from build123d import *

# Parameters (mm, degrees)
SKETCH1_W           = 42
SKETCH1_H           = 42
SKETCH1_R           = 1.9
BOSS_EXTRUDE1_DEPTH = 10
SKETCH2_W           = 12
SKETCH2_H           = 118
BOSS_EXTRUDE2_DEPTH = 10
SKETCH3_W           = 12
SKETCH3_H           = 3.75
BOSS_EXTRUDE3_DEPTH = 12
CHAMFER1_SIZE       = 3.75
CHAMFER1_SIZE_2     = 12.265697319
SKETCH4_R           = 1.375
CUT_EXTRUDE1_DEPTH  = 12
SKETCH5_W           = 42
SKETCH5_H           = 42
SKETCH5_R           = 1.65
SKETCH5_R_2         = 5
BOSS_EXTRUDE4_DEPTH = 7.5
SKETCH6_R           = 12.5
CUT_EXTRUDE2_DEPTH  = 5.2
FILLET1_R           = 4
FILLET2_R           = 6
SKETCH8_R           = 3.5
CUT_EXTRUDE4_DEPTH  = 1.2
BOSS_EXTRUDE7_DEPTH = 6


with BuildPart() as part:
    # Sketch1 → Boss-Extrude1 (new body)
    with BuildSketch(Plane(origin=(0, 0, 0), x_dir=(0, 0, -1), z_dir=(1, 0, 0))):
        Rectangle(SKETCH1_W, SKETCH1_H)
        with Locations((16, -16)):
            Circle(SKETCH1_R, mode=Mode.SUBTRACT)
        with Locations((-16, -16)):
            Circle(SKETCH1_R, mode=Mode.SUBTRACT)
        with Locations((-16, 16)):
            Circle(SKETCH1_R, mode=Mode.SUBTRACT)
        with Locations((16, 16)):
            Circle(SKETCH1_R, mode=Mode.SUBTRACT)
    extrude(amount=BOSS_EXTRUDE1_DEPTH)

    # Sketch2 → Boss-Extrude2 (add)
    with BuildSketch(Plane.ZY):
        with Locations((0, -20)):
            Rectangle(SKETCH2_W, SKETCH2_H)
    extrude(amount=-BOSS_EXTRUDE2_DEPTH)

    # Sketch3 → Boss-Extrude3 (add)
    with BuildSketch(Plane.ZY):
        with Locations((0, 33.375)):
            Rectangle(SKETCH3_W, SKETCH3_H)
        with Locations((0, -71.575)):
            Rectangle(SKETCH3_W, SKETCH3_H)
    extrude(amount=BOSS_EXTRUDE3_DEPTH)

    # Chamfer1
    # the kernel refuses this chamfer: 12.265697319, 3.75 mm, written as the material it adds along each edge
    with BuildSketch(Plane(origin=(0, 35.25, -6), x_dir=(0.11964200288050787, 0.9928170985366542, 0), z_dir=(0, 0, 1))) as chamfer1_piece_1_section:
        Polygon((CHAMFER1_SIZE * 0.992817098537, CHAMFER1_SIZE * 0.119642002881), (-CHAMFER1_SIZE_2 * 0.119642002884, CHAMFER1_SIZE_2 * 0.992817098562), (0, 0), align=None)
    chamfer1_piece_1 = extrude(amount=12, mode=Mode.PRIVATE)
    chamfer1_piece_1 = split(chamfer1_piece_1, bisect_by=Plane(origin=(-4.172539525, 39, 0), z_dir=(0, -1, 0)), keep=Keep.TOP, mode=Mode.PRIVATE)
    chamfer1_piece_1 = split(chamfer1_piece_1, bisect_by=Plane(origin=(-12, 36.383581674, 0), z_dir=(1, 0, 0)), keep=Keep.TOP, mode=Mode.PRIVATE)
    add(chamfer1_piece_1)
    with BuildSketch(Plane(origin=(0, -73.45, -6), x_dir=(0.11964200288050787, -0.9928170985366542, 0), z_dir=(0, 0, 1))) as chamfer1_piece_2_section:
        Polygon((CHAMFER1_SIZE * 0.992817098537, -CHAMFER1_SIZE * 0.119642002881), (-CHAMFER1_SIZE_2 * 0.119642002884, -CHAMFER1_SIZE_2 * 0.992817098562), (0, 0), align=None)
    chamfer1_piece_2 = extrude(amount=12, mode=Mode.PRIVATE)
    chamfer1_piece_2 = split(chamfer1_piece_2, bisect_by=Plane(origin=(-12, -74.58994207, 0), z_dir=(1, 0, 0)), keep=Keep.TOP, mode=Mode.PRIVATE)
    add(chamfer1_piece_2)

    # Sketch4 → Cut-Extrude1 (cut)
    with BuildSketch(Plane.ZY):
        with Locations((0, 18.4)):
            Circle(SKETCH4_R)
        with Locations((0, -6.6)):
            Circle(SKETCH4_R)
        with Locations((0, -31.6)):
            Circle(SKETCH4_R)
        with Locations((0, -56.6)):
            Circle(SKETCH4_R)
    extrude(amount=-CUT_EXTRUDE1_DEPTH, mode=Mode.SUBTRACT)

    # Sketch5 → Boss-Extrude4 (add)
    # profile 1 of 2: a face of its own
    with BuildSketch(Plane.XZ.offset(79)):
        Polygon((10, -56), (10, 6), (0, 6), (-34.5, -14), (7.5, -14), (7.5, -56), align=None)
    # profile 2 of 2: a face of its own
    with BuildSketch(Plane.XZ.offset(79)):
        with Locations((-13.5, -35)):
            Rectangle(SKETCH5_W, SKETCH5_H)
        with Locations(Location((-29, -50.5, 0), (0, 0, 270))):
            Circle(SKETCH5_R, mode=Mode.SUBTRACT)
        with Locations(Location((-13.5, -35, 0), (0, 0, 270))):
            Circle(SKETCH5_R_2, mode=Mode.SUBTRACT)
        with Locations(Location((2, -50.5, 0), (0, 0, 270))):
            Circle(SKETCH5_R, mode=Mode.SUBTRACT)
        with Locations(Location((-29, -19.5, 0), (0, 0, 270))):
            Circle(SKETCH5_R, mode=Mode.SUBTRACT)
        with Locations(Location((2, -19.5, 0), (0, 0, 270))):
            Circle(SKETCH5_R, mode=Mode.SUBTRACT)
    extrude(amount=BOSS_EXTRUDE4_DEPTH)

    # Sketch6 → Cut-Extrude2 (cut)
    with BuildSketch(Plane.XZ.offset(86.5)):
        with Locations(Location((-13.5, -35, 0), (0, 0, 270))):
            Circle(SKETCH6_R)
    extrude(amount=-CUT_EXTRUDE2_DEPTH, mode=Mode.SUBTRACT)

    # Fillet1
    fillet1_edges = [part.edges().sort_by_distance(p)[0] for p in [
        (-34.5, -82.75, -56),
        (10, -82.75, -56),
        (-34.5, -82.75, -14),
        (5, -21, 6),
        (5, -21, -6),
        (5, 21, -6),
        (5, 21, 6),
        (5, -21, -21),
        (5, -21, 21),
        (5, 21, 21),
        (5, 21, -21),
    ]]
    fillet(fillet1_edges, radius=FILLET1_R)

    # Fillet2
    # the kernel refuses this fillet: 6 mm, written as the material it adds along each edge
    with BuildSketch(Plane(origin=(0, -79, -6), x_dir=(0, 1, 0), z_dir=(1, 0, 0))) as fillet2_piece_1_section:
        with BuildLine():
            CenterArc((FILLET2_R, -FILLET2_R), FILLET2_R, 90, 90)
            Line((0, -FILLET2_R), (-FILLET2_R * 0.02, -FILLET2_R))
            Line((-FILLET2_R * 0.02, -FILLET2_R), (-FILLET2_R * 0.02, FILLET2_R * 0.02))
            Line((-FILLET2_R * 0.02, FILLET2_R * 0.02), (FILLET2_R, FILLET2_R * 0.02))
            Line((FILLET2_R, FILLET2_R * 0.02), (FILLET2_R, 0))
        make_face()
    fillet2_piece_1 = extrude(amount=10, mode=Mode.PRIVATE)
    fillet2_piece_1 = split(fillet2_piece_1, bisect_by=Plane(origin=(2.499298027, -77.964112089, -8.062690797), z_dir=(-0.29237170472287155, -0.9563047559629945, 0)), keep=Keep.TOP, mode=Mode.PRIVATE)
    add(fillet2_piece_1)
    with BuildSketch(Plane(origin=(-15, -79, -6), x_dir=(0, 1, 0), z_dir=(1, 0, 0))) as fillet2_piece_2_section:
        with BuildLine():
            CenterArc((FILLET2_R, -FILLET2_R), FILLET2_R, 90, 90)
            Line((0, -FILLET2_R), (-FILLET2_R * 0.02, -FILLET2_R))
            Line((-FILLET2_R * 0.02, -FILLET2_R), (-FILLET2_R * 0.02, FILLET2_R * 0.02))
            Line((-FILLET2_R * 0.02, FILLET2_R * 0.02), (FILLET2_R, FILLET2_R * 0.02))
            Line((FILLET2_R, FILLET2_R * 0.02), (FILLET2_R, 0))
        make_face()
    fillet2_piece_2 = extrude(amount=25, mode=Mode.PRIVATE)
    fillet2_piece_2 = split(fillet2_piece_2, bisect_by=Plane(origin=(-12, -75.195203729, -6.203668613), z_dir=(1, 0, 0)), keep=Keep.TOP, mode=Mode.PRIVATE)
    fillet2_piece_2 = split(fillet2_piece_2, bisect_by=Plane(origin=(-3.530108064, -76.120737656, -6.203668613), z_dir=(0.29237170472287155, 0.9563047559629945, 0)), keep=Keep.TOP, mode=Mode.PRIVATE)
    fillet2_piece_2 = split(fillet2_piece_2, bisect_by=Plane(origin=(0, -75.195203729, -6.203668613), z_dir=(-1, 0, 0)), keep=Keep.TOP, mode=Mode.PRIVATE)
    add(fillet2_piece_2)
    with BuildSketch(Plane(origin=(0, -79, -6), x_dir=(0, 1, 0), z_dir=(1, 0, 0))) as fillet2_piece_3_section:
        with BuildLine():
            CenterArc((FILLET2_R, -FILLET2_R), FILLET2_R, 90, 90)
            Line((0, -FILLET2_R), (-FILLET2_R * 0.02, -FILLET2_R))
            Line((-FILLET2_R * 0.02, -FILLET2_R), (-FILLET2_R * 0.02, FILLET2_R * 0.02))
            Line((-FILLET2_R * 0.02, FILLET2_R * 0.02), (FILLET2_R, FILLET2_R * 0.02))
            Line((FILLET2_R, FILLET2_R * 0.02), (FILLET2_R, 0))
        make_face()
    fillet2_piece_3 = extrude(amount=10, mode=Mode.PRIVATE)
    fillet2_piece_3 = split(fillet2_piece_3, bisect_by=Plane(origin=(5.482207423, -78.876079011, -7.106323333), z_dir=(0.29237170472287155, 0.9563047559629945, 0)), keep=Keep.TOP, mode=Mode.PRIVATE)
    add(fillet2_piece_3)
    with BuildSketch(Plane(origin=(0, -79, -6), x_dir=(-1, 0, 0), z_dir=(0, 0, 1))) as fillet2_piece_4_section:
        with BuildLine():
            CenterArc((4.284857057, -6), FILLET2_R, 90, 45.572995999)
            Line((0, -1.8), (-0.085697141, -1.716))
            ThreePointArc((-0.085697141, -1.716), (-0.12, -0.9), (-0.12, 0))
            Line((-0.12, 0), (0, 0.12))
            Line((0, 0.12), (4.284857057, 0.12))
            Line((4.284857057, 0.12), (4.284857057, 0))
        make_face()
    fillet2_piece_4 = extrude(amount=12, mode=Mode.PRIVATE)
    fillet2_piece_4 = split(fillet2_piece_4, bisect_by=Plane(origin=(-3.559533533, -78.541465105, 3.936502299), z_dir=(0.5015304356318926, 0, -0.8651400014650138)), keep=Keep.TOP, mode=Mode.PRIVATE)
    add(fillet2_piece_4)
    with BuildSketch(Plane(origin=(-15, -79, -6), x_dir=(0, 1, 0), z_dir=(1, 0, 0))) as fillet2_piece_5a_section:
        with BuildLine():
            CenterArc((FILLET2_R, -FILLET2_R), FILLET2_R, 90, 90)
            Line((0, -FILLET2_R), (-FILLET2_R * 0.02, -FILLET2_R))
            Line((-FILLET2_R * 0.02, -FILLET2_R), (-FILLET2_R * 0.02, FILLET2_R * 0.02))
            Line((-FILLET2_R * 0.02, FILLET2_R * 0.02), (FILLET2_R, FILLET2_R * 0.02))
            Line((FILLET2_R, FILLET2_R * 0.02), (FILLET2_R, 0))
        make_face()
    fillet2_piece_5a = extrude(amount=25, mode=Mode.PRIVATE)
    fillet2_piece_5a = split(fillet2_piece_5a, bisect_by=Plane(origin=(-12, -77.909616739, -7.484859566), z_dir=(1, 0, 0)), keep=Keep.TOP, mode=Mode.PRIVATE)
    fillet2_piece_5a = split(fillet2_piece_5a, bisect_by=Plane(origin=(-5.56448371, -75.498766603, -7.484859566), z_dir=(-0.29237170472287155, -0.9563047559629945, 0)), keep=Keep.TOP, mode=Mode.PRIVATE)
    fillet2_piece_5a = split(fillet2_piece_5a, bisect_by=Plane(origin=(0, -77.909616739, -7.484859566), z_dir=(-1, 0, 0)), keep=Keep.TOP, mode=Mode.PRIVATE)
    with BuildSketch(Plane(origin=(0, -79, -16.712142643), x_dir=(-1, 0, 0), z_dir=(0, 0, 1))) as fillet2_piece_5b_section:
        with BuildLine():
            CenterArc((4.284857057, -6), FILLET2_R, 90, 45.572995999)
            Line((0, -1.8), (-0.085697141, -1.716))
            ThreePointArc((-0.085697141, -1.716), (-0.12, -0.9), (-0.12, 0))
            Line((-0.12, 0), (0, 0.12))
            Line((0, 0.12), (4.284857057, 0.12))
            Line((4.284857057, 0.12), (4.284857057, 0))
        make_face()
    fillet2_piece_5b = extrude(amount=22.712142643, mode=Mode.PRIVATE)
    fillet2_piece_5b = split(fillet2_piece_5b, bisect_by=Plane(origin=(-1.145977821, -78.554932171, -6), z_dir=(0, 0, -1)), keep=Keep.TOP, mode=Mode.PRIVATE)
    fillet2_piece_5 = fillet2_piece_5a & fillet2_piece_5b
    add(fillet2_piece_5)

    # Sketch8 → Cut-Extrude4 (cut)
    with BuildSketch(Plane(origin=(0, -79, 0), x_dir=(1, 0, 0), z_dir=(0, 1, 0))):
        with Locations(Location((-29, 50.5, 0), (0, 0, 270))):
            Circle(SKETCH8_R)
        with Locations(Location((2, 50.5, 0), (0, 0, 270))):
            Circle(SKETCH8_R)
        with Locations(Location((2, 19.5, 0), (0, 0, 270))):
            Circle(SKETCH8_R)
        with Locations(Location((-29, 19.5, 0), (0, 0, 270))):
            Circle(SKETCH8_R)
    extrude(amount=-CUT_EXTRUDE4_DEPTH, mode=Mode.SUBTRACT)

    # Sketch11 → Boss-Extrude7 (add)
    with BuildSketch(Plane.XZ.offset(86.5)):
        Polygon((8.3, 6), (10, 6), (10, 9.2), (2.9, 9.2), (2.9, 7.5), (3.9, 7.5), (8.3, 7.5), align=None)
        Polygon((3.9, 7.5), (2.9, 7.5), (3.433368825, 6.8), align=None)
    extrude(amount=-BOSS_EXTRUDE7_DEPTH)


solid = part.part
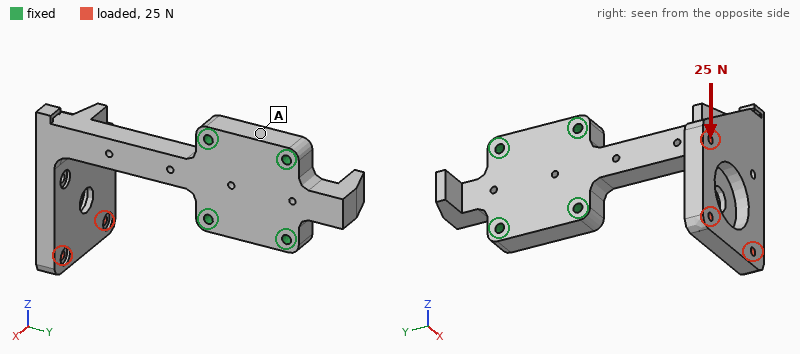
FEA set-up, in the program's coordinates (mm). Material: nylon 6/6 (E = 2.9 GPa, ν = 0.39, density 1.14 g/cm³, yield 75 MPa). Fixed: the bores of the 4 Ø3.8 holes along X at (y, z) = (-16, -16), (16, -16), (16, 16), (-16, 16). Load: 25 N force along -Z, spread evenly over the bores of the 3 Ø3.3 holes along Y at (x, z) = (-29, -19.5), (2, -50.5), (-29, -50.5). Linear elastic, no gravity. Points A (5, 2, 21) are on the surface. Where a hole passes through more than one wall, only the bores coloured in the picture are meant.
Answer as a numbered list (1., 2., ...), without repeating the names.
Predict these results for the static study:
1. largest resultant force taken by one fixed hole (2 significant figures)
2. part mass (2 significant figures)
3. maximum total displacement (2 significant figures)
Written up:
1. 53 N
2. 49 g
3. 1.7 mm
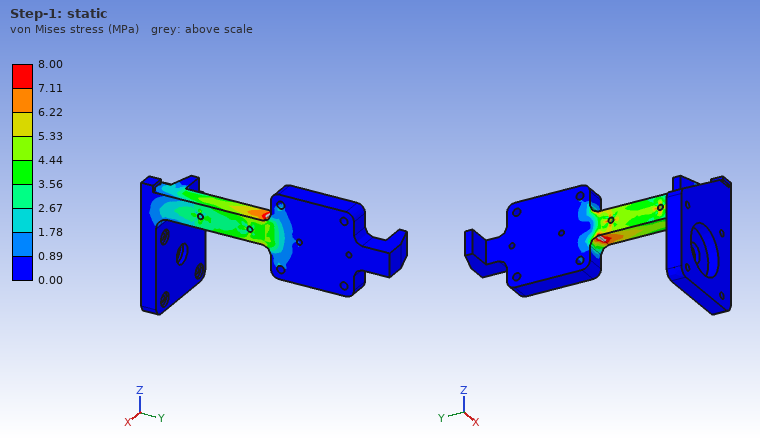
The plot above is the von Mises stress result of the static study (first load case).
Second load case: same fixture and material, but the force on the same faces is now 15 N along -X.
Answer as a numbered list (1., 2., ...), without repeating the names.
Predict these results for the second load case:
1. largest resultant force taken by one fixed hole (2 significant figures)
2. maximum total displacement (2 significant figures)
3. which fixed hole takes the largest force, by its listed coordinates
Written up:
1. 41 N
2. 1.8 mm
3. (-16, -16)
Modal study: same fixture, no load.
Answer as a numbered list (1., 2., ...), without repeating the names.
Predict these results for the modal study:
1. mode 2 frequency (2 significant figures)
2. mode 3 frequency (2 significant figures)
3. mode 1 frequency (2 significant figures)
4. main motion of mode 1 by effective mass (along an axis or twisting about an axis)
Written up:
1. 180 Hz
2. 360 Hz
3. 140 Hz
4. along X
